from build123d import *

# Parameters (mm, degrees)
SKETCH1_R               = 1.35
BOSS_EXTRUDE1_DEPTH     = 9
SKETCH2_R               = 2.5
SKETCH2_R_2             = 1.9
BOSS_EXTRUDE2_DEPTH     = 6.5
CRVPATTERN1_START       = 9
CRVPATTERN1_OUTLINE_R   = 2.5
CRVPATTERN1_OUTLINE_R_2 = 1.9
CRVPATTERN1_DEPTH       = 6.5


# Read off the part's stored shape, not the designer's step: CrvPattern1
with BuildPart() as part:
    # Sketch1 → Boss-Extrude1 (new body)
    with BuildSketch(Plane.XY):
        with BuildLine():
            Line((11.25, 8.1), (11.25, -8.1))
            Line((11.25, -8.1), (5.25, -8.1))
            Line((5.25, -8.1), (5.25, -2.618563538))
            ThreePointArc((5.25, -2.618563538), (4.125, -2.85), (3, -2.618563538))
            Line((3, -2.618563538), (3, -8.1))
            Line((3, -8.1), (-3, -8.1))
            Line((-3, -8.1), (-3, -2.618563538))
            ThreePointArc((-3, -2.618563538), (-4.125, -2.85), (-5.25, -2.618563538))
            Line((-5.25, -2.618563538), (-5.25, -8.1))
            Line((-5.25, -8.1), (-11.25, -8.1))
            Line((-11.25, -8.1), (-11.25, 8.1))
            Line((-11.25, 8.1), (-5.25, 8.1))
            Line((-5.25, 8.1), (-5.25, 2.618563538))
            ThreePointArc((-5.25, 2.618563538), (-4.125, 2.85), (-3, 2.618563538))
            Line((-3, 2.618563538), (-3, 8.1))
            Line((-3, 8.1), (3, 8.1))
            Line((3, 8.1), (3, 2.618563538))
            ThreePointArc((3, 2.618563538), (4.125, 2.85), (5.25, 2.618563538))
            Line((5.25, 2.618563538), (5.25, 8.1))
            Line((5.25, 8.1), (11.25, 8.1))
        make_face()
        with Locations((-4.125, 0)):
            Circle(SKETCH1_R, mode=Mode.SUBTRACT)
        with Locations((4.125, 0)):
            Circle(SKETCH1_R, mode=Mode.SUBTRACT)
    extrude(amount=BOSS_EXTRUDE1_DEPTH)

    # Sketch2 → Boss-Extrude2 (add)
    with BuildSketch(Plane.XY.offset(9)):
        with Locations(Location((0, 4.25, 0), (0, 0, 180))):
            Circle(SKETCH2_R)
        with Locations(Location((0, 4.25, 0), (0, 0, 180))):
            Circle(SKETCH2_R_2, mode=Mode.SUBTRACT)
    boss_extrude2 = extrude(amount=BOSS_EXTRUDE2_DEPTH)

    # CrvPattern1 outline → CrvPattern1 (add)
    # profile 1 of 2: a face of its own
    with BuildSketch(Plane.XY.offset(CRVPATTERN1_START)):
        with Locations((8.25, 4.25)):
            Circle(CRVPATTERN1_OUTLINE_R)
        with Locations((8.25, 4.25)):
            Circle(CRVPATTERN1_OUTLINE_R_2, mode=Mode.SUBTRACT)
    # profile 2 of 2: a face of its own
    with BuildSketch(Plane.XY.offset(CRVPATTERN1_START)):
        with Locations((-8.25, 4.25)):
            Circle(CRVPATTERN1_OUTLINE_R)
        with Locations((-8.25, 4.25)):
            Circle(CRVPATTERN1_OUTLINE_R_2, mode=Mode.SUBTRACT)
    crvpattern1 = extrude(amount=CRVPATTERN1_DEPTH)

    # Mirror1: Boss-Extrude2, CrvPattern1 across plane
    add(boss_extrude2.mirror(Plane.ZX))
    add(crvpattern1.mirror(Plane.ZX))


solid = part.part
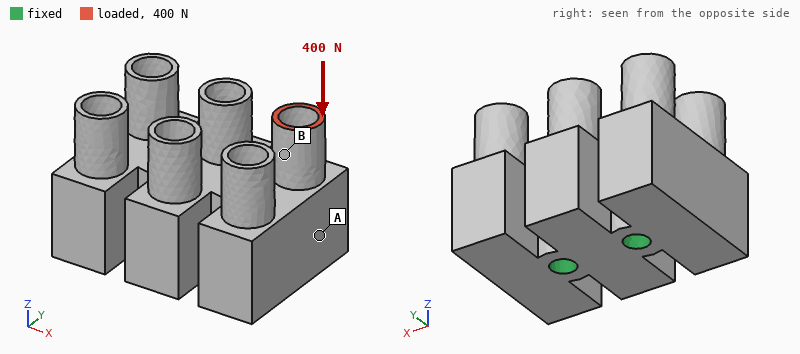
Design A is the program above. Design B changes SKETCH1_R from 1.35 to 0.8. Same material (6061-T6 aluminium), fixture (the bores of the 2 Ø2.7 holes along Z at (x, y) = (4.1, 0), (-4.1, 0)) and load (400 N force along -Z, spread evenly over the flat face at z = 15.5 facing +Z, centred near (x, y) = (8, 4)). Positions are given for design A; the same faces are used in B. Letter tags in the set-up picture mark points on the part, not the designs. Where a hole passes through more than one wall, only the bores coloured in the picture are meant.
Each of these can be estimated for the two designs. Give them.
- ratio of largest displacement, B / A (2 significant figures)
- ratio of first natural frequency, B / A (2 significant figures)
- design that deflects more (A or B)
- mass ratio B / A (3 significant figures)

1.2
0.84
B
1.02
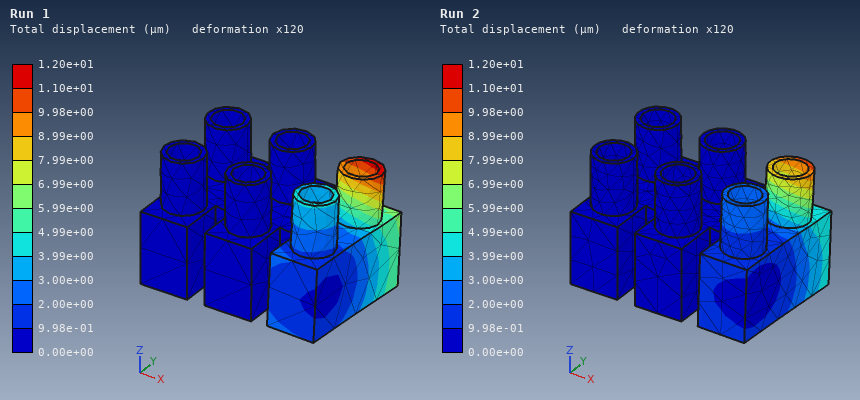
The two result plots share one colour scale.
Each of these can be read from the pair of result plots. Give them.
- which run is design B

Run 1
